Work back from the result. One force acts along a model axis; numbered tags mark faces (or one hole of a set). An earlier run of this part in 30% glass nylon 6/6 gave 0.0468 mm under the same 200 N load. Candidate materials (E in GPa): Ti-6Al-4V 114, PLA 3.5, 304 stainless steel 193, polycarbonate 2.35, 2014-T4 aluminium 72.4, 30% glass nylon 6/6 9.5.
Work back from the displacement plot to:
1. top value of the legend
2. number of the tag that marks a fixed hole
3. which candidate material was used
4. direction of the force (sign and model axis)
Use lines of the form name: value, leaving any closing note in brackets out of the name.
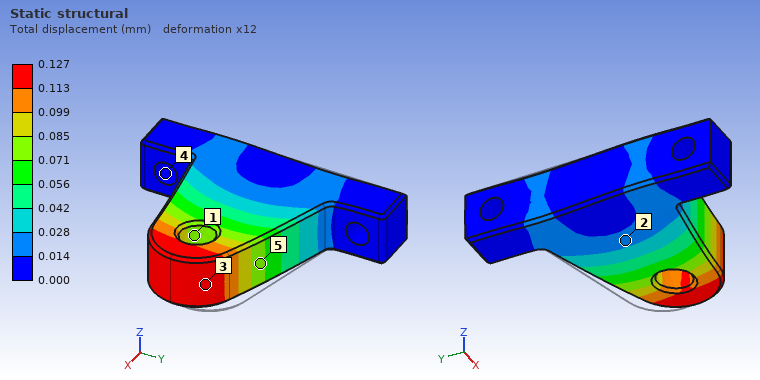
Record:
top value of the legend: 0.127 mm
number of the tag that marks a fixed hole: 4
which candidate material was used: PLA
direction of the force: -Y
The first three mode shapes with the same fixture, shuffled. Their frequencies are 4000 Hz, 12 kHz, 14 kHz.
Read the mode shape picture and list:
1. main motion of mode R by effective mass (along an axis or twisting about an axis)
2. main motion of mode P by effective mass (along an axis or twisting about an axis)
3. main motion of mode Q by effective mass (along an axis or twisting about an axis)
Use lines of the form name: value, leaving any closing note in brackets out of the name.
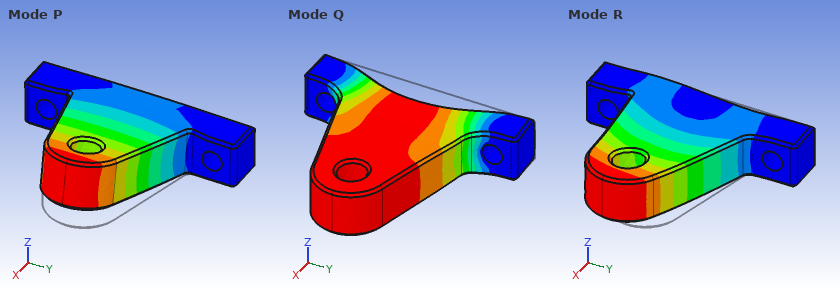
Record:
main motion of mode R by effective mass: along Y
main motion of mode P by effective mass: along Z
main motion of mode Q by effective mass: along X
